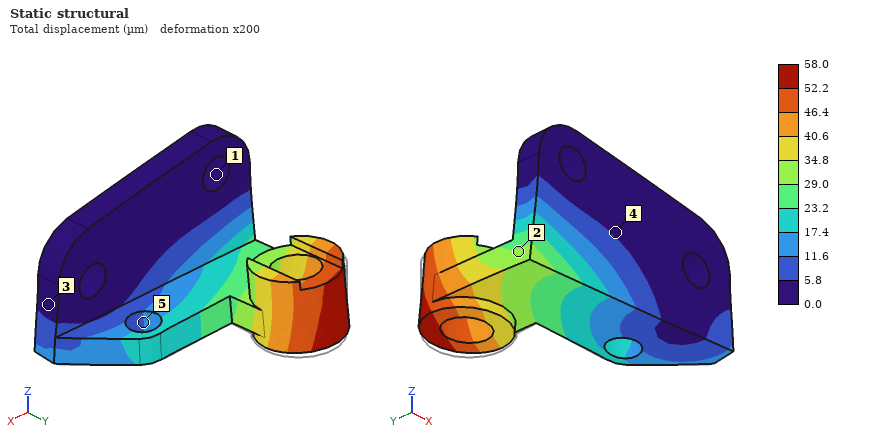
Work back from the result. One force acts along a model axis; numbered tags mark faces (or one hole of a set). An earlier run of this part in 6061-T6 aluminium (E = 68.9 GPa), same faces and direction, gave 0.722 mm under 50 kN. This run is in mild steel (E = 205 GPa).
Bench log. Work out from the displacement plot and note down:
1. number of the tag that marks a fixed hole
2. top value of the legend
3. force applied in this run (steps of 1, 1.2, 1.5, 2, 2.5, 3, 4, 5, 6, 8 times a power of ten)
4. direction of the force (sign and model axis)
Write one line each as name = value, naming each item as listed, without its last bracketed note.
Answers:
number of the tag that marks a fixed hole = 1
top value of the legend = 58.0 µm
force applied in this run = 12 kN
direction of the force = +X
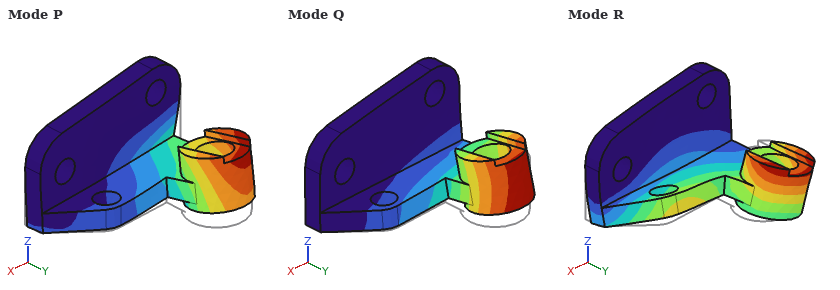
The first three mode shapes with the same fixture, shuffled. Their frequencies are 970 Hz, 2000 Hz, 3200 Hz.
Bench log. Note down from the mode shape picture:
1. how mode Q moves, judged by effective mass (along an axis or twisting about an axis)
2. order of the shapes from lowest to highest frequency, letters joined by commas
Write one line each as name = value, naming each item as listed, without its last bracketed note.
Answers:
how mode Q moves, judged by effective mass = along Z
order of the shapes from lowest to highest frequency, letters joined by commas = Q, P, R
